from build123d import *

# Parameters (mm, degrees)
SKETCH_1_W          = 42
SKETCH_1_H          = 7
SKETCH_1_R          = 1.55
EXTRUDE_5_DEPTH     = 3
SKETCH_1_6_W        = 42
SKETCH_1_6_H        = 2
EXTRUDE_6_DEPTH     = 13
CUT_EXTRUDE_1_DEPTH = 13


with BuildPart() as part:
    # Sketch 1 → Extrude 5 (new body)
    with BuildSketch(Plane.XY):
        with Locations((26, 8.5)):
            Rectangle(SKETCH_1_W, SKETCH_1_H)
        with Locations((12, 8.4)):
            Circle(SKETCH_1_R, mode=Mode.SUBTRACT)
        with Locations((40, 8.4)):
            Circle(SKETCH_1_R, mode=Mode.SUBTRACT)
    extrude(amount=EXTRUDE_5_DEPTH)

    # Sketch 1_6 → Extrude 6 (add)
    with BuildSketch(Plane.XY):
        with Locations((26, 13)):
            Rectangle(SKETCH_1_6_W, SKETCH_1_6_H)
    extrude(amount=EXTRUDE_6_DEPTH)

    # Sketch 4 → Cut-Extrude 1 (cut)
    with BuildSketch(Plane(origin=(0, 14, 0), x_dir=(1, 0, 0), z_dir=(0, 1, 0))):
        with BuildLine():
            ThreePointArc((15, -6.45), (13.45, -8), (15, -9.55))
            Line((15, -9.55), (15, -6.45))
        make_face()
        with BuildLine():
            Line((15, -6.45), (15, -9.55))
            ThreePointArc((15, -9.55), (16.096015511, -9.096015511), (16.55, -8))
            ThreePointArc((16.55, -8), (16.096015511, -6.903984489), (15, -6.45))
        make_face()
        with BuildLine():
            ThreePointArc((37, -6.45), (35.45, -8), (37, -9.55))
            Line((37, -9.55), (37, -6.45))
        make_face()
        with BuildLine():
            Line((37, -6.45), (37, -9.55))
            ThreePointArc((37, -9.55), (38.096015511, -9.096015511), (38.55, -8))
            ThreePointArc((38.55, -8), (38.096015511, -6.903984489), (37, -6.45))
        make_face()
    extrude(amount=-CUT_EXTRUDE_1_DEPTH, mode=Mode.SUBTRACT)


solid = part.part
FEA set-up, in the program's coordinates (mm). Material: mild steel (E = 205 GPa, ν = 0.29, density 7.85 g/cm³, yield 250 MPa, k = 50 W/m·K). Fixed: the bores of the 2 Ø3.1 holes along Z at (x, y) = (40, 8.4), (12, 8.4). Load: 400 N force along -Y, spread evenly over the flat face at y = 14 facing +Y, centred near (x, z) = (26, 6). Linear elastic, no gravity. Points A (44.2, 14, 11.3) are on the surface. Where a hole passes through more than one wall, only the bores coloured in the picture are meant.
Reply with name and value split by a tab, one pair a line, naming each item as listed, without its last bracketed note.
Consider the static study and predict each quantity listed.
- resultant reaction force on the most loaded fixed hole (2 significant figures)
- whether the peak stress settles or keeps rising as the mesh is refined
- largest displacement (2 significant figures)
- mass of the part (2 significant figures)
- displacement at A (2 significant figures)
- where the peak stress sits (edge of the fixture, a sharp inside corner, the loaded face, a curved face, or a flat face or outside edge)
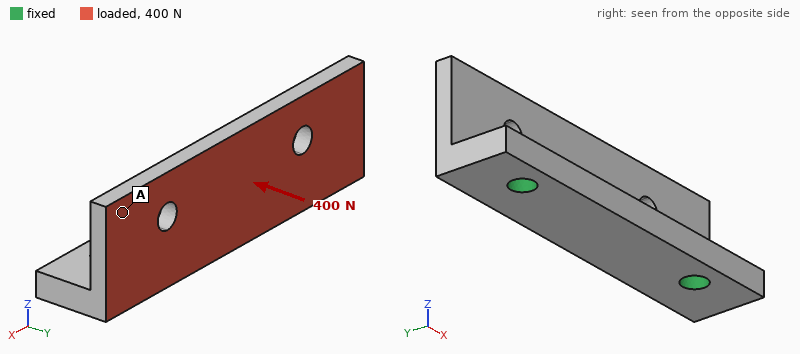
resultant reaction force on the most loaded fixed hole	200 N
whether the peak stress settles or keeps rising as the mesh is refined	keeps rising
largest displacement	18 µm
mass of the part	15 g
displacement at A	13 µm
where the peak stress sits	edge of the fixture
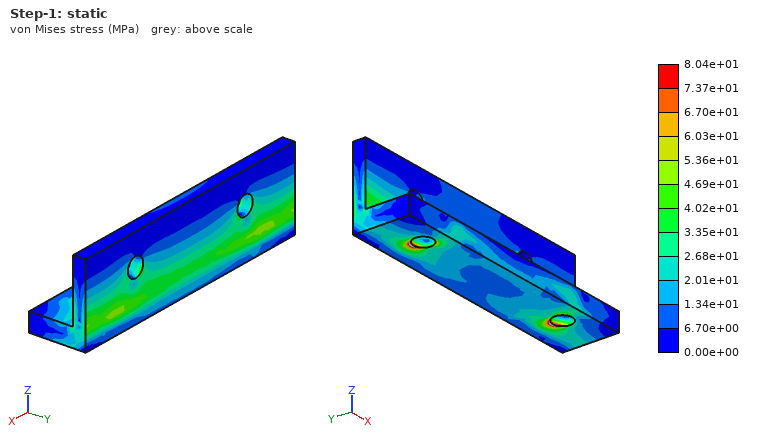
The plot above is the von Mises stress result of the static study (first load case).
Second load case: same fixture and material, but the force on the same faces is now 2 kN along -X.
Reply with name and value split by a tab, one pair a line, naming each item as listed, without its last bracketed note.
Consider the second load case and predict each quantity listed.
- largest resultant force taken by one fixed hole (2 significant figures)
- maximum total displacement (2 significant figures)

largest resultant force taken by one fixed hole	1.1 kN
maximum total displacement	7.8 µm
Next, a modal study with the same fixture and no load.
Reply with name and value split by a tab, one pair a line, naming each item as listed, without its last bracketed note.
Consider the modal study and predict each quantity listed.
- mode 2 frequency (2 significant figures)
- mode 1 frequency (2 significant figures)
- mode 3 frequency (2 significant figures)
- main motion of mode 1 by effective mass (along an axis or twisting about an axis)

mode 2 frequency	13 kHz
mode 1 frequency	10 kHz
mode 3 frequency	18 kHz
main motion of mode 1 by effective mass	along Y
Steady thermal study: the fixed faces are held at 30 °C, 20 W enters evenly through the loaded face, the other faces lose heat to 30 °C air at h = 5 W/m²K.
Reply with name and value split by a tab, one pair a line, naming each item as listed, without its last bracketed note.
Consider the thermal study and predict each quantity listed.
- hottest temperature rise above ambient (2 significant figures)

hottest temperature rise above ambient	51 K
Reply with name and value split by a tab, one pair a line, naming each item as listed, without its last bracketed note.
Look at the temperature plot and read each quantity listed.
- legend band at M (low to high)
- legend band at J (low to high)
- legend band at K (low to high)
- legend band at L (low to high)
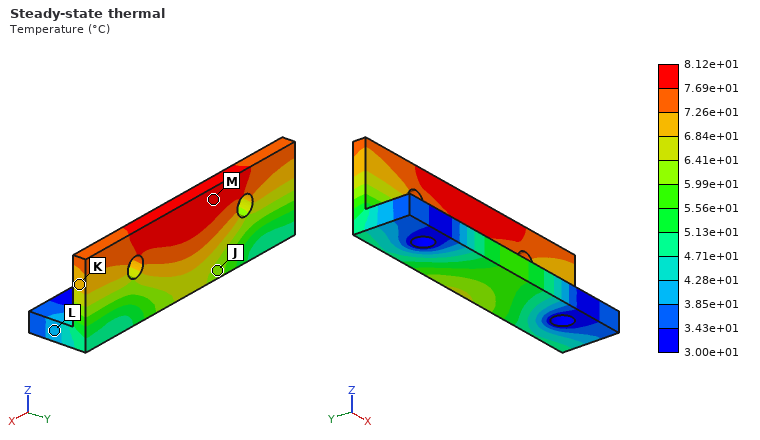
legend band at M	7.69e+01 to 8.12e+01 °C
legend band at J	5.99e+01 to 6.41e+01 °C
legend band at K	6.84e+01 to 7.26e+01 °C
legend band at L	3.85e+01 to 4.28e+01 °C
